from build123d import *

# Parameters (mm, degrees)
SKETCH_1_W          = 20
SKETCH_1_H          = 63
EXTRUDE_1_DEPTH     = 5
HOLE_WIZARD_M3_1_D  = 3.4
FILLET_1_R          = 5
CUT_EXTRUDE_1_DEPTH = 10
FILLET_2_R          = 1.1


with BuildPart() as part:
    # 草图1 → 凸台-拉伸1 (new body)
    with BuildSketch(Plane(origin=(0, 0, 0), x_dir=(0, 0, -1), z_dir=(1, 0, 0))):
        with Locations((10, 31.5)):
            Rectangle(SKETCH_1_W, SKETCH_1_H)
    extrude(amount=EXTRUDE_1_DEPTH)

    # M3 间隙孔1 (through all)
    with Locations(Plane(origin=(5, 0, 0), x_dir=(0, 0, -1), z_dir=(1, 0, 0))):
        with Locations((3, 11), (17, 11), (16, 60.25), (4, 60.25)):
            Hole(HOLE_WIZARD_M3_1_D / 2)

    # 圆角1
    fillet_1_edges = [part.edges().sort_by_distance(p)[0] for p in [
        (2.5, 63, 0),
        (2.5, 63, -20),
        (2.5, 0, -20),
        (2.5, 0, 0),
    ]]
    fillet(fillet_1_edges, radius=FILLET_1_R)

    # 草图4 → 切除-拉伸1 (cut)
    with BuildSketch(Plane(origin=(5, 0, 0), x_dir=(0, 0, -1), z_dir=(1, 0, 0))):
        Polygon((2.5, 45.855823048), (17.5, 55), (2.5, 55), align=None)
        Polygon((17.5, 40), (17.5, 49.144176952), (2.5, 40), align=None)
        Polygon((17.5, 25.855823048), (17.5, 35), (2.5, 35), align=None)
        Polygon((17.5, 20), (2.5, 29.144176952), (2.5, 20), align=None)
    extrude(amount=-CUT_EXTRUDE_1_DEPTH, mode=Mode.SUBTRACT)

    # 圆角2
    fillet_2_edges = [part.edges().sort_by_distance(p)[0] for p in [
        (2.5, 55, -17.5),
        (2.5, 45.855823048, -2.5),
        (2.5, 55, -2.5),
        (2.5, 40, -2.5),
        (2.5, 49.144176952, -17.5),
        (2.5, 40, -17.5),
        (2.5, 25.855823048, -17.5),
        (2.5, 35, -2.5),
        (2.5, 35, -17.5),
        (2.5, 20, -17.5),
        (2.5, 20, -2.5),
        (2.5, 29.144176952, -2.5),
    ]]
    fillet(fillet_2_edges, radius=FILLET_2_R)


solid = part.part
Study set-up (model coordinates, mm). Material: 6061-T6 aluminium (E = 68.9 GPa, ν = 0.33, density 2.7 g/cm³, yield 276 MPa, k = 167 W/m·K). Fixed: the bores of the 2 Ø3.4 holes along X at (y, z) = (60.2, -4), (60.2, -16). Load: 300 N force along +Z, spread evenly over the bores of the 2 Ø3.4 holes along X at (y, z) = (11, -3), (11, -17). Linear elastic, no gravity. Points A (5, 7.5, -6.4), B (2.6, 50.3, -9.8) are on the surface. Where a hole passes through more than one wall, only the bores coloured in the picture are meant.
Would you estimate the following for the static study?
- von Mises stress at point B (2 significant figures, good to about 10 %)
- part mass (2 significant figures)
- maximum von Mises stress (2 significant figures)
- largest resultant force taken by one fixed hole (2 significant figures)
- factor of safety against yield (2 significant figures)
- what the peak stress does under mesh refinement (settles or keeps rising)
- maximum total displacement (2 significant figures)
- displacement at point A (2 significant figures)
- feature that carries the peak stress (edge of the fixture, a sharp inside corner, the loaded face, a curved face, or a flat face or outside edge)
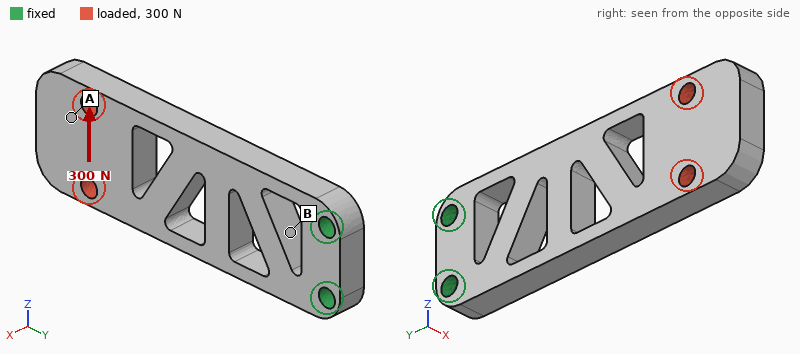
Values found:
22 MPa
13 g
100 MPa
980 N
2.7
settles
0.14 mm
0.12 mm
a curved face
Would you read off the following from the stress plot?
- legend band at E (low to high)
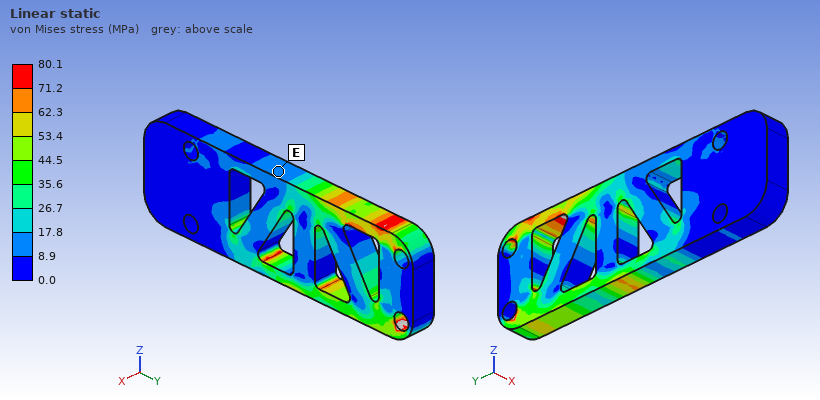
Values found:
8.9 to 17.8 MPa
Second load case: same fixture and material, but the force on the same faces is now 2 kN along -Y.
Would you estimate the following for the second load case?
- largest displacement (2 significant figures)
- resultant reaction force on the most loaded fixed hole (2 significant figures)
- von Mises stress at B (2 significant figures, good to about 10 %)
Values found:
42 µm
1.1 kN
16 MPa
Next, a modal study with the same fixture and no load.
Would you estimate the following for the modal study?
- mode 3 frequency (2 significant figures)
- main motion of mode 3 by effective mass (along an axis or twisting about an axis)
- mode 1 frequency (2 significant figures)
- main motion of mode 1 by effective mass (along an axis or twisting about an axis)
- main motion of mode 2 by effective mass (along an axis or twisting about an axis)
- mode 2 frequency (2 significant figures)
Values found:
4700 Hz
twisting about Y
810 Hz
along X
along Z
3300 Hz
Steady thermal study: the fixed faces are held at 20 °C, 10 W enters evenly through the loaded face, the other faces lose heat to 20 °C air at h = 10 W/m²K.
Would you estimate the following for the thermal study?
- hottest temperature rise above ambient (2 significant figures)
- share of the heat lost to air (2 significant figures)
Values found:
58 K
11 %
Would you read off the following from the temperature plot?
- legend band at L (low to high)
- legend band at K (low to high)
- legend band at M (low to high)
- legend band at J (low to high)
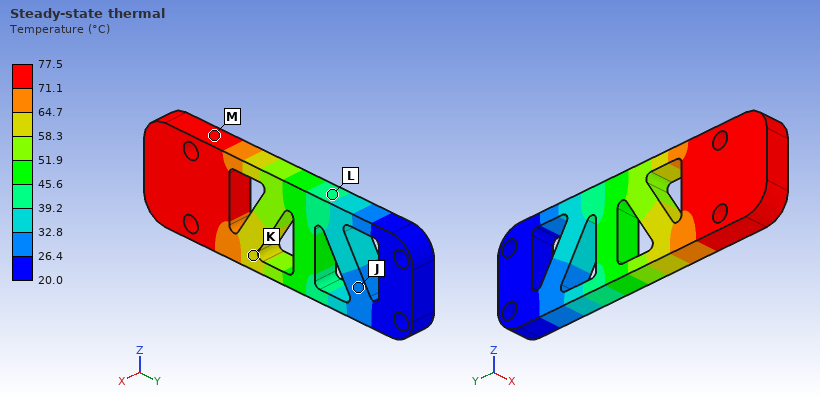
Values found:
39.2 to 45.6 °C
58.3 to 64.7 °C
71.1 to 77.5 °C
26.4 to 32.8 °C
